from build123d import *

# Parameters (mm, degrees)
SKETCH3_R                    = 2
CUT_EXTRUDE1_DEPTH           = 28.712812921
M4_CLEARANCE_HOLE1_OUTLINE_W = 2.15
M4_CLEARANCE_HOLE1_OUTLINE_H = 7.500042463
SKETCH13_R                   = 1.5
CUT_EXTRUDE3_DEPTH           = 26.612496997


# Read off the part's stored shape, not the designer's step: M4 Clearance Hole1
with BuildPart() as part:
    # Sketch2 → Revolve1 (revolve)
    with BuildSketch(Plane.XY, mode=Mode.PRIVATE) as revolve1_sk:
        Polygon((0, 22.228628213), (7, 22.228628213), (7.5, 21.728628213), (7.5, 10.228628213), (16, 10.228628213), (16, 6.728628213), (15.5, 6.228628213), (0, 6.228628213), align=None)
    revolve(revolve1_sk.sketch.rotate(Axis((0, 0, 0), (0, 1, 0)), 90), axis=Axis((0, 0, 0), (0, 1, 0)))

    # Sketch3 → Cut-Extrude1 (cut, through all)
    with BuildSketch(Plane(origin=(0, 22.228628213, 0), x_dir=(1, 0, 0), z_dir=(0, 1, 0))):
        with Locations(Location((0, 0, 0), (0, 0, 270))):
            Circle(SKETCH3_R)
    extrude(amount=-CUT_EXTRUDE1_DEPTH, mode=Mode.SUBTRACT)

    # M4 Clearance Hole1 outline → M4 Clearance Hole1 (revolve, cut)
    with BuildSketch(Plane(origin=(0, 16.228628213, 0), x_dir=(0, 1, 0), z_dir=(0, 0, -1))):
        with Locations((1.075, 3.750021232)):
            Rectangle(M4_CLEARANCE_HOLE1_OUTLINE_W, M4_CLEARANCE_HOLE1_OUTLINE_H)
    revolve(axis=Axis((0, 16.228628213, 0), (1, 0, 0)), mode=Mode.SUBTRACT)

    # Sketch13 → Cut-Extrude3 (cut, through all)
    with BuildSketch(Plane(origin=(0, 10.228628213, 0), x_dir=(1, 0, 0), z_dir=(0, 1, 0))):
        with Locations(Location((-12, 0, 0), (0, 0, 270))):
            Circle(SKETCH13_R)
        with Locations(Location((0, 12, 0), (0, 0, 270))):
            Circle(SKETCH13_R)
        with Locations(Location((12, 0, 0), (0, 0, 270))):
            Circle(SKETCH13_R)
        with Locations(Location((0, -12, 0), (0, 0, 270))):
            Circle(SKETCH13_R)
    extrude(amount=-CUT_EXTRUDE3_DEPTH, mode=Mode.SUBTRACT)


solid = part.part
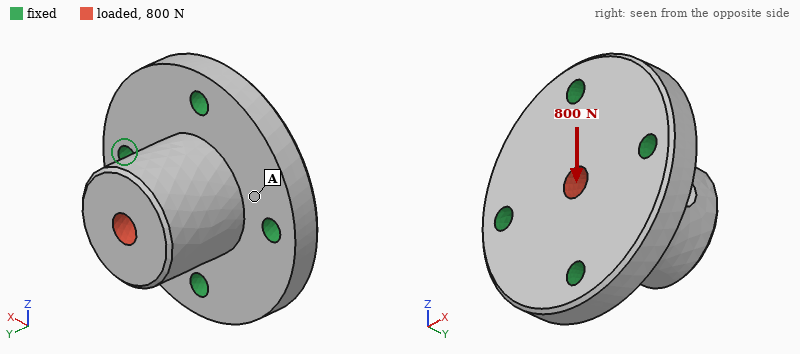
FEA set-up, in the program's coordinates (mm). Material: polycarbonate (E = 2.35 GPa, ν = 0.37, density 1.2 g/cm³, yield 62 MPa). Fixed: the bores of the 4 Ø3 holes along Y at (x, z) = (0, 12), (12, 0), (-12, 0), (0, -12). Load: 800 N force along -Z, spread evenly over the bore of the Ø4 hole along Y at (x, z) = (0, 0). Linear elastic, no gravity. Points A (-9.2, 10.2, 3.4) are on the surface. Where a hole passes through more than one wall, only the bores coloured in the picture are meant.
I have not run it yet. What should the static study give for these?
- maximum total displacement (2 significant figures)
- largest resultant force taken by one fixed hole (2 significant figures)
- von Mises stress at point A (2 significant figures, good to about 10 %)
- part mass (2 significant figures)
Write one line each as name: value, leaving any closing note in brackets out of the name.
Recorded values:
maximum total displacement: 0.18 mm
largest resultant force taken by one fixed hole: 340 N
von Mises stress at point A: 4.8 MPa
part mass: 5.9 g
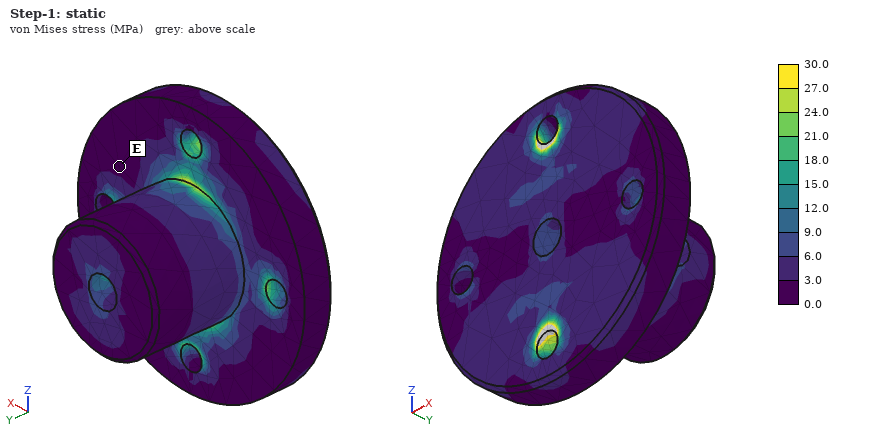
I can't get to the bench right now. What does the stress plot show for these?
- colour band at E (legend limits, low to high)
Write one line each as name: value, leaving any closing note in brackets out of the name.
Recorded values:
colour band at E: 0.0 to 3.0 MPa
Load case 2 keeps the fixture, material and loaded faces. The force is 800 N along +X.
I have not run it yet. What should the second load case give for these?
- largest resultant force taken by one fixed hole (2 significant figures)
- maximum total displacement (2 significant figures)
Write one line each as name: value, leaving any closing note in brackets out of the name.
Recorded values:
largest resultant force taken by one fixed hole: 350 N
maximum total displacement: 0.18 mm
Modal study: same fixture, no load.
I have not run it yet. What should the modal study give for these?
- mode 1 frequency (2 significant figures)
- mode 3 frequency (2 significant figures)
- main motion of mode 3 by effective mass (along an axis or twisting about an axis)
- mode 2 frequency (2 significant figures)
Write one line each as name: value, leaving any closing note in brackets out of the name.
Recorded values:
mode 1 frequency: 7000 Hz
mode 3 frequency: 9400 Hz
main motion of mode 3 by effective mass: along Y
mode 2 frequency: 7100 Hz
